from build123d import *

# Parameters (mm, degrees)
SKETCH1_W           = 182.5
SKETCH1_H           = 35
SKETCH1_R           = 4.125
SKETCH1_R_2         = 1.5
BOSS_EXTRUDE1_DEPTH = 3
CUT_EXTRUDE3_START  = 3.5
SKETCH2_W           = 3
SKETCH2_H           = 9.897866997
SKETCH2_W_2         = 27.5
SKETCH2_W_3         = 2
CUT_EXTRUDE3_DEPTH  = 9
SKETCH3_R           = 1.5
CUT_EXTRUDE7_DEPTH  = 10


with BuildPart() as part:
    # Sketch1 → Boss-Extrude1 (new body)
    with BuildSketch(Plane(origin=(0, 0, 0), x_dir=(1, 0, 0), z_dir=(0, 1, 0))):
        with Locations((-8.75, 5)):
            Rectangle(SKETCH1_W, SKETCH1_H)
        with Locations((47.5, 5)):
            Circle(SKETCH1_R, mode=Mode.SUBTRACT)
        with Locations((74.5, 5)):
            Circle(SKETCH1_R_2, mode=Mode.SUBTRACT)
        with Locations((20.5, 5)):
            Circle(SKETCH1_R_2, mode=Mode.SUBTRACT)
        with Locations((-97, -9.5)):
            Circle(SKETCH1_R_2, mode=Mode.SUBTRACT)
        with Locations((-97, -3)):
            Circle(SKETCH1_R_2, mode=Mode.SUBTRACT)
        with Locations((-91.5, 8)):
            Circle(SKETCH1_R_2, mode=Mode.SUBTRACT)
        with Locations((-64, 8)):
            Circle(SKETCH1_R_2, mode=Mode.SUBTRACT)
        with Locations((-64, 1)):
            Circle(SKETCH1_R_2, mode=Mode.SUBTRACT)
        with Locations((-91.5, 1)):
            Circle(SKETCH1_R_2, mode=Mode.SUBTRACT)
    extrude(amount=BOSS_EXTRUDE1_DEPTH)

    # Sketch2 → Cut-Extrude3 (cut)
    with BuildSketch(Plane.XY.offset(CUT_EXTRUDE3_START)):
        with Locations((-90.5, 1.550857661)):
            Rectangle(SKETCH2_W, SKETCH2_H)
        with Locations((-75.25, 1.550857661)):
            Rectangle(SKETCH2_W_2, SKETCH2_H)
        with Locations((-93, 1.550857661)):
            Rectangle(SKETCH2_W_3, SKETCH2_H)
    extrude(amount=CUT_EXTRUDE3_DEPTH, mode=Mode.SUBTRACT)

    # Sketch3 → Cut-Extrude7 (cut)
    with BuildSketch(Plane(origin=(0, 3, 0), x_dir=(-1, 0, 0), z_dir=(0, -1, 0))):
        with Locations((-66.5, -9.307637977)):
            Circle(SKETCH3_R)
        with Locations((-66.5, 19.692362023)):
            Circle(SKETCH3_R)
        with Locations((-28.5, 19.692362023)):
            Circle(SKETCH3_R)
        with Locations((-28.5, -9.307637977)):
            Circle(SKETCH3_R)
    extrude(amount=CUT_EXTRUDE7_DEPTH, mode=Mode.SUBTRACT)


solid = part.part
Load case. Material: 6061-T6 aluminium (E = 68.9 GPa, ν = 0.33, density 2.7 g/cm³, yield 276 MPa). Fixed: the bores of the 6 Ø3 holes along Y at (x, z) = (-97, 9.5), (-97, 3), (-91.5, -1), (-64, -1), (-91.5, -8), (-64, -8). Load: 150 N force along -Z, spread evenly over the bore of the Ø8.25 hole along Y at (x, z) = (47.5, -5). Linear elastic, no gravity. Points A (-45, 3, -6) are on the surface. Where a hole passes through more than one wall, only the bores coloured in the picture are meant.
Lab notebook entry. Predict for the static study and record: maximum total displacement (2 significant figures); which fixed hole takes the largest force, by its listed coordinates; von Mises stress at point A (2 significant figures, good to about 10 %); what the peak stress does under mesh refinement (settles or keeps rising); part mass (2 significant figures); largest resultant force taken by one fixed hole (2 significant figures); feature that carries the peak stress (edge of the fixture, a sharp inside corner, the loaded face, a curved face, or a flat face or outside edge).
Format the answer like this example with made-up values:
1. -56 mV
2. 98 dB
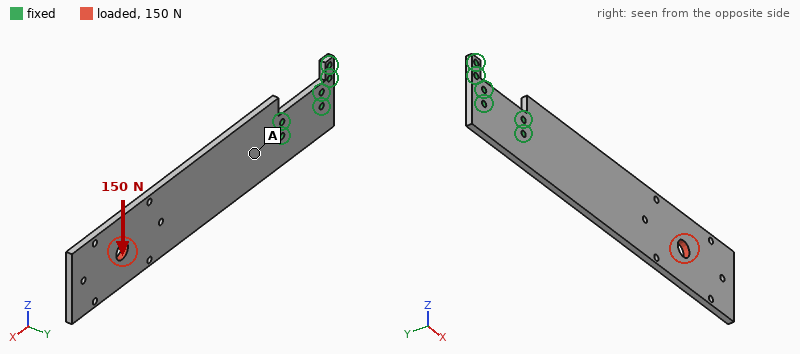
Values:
1. 0.26 mm
2. (-64, -1)
3. 7.0 MPa
4. keeps rising
5. 48 g
6. 980 N
7. edge of the fixture
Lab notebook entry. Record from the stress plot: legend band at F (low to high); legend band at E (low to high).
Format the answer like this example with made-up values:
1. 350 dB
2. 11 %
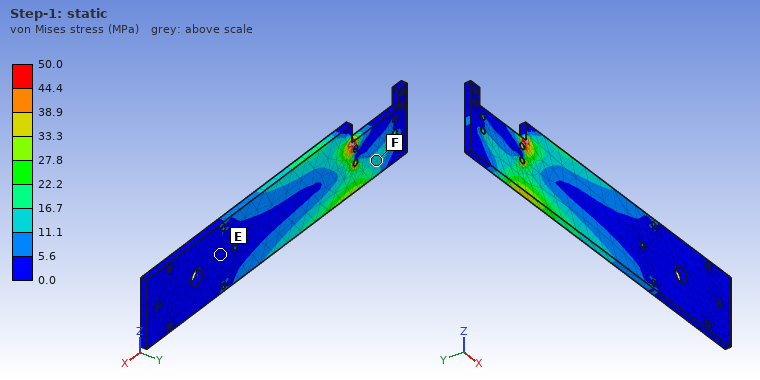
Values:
1. 11.1 to 16.7 MPa
2. 0.0 to 5.6 MPa
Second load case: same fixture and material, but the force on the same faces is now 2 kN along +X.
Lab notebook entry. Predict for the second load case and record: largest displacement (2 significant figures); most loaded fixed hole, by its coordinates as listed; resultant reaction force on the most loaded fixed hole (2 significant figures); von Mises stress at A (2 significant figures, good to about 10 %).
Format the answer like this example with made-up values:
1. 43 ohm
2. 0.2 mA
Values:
1. 51 µm
2. (-64, -1)
3. 1.0 kN
4. 24 MPa
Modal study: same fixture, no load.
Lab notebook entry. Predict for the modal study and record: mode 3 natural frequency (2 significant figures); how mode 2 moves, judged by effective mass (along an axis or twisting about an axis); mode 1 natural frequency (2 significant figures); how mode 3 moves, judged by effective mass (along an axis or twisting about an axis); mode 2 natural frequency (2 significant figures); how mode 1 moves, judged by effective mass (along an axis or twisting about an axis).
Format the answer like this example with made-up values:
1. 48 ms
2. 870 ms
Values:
1. 890 Hz
2. along Y
3. 110 Hz
4. twisting about X
5. 700 Hz
6. along Y
